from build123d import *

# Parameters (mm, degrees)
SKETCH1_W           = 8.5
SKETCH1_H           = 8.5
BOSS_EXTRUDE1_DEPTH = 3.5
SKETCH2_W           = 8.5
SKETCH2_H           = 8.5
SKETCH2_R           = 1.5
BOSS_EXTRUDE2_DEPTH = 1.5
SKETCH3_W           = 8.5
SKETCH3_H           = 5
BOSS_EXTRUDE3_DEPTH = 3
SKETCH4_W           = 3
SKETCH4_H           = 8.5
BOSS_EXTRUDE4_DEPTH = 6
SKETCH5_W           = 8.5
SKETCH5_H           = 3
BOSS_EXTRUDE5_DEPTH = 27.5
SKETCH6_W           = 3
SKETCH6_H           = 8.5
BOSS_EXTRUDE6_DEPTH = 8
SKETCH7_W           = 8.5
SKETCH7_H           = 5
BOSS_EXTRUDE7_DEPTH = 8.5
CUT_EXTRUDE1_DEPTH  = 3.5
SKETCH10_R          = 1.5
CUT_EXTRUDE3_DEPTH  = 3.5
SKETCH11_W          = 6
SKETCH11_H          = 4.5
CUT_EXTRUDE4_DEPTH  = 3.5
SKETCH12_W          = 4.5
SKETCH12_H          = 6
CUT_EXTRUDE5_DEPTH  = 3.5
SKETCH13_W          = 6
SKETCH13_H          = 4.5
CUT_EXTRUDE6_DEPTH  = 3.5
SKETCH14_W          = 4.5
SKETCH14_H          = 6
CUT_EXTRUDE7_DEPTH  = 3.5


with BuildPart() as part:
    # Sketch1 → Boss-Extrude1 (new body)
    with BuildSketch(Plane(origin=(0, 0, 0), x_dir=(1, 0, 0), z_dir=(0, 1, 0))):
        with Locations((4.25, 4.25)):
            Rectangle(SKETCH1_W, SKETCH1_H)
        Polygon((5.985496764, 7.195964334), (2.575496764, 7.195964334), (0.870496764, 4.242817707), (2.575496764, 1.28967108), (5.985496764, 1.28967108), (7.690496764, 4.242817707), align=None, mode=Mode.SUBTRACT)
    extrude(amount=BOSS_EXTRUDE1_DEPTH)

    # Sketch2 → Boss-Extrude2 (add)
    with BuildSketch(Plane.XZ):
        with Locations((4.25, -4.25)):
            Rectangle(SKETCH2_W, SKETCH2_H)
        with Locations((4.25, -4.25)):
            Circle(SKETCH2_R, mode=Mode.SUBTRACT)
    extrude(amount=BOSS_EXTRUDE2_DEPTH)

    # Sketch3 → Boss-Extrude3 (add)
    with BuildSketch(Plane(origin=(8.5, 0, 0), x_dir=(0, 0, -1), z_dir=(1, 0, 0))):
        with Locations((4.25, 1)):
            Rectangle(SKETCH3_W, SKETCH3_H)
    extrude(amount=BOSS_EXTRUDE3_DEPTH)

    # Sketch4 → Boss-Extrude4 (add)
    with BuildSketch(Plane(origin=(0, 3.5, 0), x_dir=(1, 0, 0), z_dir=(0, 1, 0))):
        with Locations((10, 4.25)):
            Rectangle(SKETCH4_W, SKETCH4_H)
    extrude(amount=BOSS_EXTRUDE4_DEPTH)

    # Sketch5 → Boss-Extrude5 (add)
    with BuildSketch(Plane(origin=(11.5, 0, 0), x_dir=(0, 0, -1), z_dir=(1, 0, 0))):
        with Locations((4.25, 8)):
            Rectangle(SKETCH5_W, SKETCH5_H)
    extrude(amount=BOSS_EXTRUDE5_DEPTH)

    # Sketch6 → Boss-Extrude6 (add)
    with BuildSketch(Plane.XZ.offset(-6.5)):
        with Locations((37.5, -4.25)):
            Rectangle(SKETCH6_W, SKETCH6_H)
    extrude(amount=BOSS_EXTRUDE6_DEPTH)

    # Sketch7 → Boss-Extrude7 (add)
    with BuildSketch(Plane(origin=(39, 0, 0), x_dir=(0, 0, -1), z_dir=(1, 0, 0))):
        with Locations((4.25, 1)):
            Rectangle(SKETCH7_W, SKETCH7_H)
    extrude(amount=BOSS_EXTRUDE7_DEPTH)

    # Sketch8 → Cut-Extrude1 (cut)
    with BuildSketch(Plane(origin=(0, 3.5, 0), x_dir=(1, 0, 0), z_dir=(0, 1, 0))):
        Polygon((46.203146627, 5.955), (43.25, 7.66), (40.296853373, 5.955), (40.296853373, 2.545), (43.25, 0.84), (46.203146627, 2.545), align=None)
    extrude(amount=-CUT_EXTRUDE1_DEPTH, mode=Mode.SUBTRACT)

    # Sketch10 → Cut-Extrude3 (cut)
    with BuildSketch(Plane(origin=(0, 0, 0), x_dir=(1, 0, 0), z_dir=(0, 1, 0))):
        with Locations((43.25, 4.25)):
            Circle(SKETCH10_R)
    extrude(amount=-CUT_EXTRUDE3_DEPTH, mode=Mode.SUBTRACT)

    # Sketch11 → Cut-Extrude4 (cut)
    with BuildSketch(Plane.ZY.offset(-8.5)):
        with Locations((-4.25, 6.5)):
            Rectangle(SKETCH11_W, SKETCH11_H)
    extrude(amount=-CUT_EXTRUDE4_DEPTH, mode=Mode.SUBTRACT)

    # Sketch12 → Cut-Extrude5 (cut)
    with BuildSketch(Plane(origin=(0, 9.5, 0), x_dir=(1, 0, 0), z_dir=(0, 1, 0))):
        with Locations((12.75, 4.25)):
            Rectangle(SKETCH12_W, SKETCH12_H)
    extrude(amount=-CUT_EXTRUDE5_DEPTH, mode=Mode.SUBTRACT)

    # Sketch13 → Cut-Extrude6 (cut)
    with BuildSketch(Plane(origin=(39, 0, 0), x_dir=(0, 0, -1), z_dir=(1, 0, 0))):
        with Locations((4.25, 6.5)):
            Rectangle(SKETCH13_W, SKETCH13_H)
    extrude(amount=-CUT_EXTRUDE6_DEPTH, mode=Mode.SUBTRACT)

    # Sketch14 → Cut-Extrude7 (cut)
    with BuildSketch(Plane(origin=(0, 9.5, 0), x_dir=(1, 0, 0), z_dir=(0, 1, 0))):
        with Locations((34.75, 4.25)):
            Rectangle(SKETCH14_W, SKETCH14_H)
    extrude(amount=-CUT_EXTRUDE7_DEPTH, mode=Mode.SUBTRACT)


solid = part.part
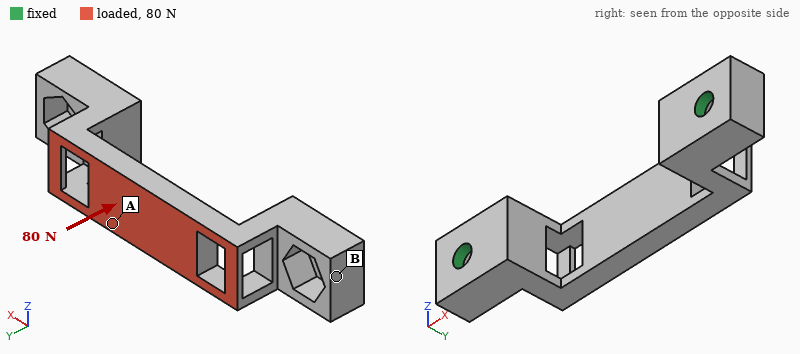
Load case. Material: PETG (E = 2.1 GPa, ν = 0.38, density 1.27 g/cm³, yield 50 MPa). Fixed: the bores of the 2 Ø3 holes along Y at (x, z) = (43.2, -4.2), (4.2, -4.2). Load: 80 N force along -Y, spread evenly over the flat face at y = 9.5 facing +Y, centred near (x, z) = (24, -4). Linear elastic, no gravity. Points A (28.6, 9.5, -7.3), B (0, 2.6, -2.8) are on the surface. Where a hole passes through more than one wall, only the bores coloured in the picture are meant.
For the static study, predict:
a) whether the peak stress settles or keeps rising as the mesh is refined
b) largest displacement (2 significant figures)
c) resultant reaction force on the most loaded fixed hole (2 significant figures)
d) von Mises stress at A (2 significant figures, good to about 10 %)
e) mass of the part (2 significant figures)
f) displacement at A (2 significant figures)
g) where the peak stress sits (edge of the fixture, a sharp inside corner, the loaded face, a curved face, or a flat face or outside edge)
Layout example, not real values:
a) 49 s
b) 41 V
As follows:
a) keeps rising
b) 0.32 mm
c) 52 N
d) 11 MPa
e) 1.8 g
f) 0.27 mm
g) a sharp inside corner
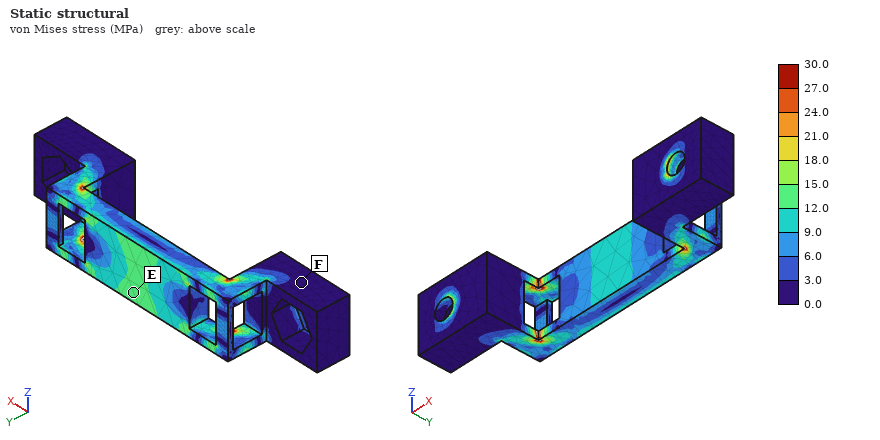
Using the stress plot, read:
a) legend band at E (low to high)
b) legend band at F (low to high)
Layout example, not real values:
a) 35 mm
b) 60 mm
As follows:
a) 12.0 to 15.0 MPa
b) 0.0 to 3.0 MPa
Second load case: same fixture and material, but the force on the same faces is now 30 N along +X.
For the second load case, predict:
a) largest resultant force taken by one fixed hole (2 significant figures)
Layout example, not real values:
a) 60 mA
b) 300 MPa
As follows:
a) 16 N
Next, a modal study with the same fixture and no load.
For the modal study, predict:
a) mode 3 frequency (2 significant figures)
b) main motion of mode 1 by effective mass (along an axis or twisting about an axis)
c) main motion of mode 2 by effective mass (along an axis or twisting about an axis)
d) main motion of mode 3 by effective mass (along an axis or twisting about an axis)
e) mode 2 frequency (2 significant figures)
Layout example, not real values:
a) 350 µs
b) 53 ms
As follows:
a) 3100 Hz
b) along Z
c) along X
d) along Y
e) 2800 Hz
